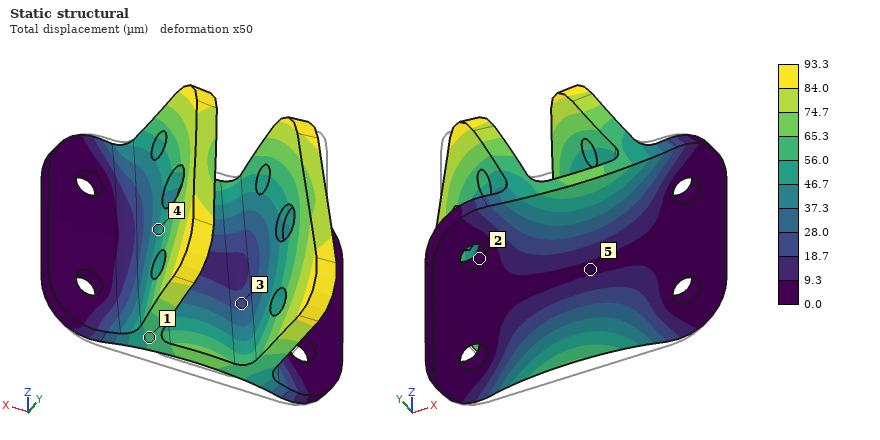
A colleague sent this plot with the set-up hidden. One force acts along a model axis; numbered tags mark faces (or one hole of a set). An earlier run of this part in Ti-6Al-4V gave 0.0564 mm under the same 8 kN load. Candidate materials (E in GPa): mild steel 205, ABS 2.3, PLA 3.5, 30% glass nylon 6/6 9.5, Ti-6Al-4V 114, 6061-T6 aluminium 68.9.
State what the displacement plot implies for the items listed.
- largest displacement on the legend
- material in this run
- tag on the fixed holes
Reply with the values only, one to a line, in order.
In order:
93.3 µm
6061-T6 aluminium
2
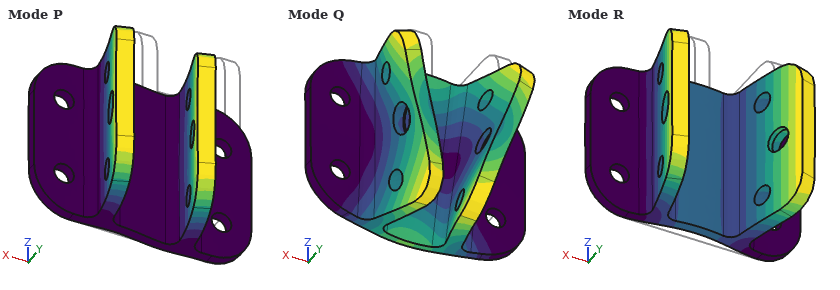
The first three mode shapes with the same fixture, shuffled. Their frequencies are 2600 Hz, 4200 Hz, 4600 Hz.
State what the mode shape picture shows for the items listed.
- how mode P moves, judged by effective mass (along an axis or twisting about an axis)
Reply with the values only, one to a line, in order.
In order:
along X
